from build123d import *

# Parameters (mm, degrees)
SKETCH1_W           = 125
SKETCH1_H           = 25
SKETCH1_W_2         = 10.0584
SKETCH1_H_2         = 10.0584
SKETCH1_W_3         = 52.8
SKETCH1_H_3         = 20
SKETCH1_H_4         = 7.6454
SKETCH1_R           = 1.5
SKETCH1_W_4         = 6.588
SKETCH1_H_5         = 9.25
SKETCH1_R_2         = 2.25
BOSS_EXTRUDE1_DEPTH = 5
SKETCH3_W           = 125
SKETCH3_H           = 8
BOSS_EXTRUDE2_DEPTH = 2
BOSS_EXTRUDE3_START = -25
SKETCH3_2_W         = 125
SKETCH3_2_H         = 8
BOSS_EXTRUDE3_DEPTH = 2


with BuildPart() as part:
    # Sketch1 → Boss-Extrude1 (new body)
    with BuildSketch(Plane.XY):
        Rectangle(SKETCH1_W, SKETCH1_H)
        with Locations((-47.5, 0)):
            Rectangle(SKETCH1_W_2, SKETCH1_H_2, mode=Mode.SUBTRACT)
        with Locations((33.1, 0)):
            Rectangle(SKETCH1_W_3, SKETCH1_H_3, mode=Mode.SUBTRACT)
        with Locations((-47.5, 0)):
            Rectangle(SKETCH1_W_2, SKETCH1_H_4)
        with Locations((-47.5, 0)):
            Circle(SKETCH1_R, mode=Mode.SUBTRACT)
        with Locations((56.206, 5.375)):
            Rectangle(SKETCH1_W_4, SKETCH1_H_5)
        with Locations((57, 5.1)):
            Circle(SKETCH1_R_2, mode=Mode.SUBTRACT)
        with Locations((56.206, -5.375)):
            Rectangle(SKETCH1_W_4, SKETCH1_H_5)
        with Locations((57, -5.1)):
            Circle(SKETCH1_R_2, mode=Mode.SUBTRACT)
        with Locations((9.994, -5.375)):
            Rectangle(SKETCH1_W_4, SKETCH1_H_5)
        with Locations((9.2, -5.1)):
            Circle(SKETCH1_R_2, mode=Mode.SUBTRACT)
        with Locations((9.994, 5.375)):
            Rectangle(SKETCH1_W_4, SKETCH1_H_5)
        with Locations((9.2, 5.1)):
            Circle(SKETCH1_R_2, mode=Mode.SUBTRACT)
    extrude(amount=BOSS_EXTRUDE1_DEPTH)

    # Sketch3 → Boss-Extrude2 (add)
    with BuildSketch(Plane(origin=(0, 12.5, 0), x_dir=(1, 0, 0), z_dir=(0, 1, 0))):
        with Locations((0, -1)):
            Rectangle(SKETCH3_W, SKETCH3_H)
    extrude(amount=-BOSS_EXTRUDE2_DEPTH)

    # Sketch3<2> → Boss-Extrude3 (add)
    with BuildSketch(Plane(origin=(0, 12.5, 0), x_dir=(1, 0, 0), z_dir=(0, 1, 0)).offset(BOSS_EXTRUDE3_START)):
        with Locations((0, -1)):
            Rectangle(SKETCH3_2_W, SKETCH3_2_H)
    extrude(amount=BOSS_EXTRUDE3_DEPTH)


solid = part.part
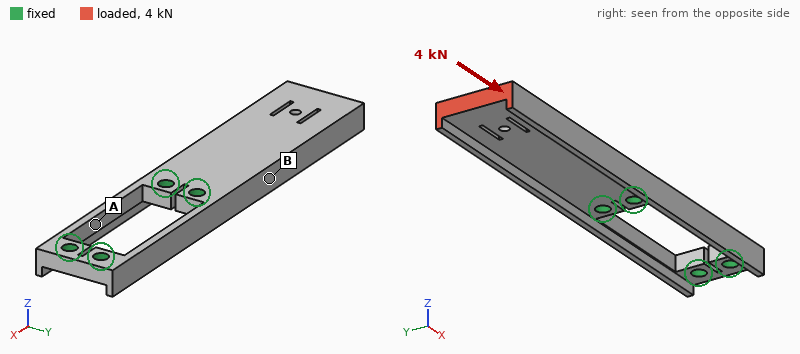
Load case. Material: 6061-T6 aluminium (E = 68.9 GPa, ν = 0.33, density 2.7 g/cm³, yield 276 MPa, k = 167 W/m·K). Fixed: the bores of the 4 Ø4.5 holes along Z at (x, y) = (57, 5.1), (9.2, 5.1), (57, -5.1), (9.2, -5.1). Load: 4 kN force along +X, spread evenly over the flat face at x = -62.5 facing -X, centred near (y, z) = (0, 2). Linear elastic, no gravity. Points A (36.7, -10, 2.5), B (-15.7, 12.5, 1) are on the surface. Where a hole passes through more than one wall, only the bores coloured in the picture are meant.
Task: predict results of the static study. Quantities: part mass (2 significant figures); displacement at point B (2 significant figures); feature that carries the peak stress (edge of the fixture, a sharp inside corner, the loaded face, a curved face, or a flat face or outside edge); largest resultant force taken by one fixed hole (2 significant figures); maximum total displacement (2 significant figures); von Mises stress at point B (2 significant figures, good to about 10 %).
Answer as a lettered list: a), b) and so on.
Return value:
a) 34 g
b) 13 µm
c) a curved face
d) 1.9 kN
e) 39 µm
f) 29 MPa
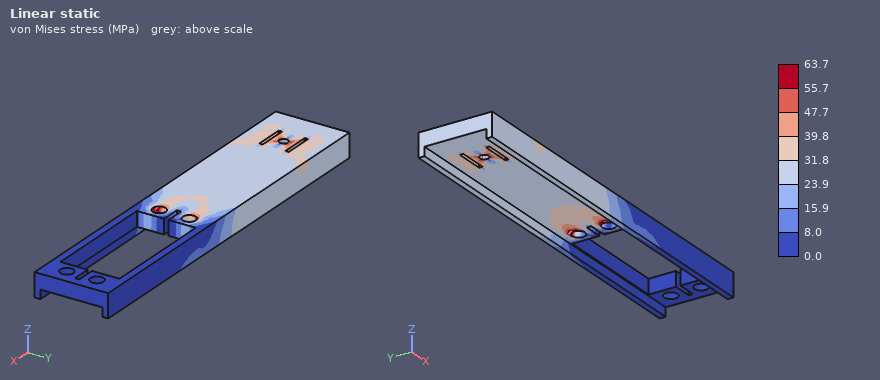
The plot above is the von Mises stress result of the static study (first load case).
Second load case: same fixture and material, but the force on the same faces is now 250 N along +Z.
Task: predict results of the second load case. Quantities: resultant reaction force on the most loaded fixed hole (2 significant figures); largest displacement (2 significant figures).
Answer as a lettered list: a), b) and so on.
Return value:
a) 260 N
b) 1.0 mm
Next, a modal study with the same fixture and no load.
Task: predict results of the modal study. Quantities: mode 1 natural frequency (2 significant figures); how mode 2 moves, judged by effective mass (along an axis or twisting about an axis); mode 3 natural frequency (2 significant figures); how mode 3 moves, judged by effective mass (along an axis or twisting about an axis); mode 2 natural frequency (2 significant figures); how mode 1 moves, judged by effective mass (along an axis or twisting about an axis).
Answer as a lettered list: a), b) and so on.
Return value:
a) 990 Hz
b) along Y
c) 4000 Hz
d) twisting about X
e) 3400 Hz
f) along Z
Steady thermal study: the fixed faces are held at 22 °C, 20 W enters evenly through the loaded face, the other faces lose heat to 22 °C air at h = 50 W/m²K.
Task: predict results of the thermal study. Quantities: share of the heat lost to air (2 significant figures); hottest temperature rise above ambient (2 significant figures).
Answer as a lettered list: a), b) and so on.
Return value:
a) 32 %
b) 50 K
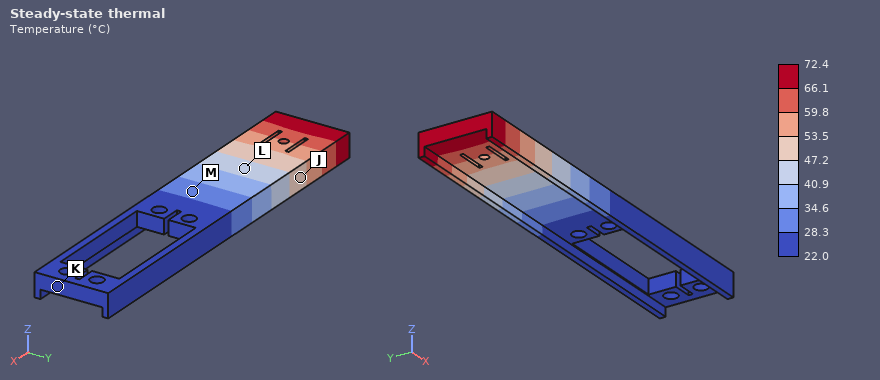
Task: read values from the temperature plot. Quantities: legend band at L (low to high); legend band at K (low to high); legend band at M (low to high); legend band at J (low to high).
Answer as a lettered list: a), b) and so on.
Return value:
a) 40.9 to 47.2 °C
b) 22.0 to 28.3 °C
c) 28.3 to 34.6 °C
d) 47.2 to 53.5 °C
